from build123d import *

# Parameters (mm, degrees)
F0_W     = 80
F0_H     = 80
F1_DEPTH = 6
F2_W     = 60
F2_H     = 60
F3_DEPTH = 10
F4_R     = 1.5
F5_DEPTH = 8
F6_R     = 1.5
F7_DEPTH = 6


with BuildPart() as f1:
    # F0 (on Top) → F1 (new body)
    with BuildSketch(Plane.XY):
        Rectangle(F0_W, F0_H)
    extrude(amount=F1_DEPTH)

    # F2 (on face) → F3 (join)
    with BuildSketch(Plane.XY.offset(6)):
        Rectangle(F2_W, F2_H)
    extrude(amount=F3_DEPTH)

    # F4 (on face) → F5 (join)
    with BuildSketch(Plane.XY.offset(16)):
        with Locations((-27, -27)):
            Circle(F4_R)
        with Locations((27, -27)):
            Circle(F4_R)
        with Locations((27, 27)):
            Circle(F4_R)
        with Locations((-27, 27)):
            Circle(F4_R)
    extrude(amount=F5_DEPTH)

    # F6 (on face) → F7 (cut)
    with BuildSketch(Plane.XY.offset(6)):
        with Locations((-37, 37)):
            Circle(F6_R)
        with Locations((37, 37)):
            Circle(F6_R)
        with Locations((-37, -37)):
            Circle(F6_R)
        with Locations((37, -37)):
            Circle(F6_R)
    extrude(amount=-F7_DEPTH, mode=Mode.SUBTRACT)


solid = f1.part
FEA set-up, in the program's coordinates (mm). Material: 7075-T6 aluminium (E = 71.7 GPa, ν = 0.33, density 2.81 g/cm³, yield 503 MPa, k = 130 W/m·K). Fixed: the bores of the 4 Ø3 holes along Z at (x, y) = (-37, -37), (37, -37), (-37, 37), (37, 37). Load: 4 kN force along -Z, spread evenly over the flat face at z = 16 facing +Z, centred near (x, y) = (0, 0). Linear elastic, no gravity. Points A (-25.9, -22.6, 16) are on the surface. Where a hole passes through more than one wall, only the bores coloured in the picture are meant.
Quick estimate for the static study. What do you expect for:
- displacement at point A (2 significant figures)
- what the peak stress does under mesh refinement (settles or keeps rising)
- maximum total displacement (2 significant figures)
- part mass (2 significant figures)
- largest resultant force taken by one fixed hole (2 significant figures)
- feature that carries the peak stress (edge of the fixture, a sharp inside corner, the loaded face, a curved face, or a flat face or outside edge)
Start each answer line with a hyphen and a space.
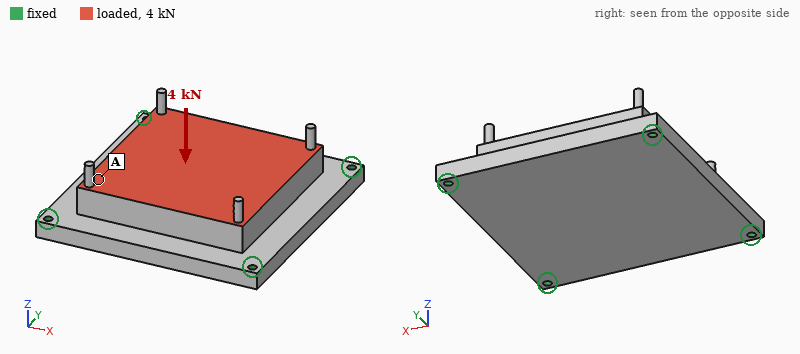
- 28 µm
- keeps rising
- 36 µm
- 210 g
- 1.2 kN
- edge of the fixture
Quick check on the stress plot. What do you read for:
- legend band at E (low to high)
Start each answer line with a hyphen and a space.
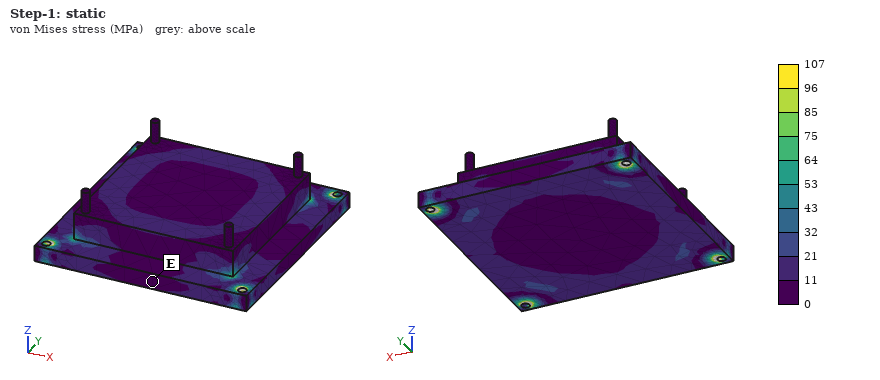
- 0 to 11 MPa
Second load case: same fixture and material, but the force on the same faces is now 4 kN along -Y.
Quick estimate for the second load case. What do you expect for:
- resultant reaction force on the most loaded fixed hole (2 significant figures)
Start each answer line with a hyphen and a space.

- 1.2 kN
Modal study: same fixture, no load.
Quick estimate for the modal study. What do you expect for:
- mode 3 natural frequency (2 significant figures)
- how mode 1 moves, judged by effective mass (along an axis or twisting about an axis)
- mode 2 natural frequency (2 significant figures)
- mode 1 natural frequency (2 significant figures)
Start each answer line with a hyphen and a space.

- 6900 Hz
- along Z
- 6900 Hz
- 4000 Hz
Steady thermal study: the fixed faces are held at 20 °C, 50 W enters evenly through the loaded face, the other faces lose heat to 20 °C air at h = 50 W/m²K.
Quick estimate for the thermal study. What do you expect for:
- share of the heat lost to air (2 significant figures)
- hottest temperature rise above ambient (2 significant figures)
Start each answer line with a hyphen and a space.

- 17 %
- 17 K
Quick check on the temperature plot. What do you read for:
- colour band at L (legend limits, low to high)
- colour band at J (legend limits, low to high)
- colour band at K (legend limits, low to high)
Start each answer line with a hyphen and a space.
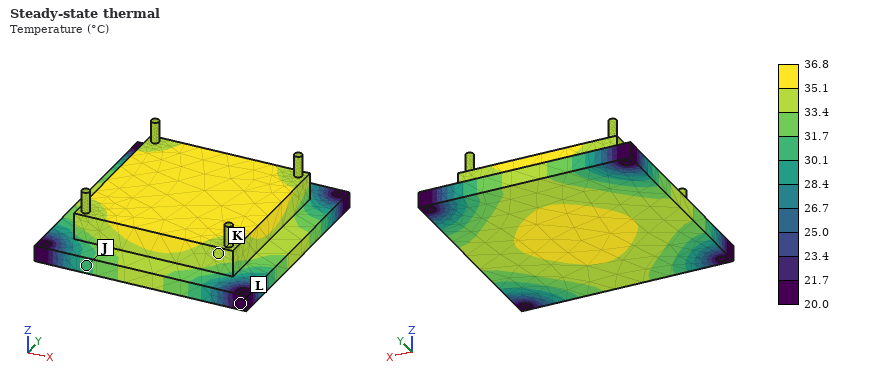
- 20.0 to 21.7 °C
- 30.1 to 31.7 °C
- 33.4 to 35.1 °C
